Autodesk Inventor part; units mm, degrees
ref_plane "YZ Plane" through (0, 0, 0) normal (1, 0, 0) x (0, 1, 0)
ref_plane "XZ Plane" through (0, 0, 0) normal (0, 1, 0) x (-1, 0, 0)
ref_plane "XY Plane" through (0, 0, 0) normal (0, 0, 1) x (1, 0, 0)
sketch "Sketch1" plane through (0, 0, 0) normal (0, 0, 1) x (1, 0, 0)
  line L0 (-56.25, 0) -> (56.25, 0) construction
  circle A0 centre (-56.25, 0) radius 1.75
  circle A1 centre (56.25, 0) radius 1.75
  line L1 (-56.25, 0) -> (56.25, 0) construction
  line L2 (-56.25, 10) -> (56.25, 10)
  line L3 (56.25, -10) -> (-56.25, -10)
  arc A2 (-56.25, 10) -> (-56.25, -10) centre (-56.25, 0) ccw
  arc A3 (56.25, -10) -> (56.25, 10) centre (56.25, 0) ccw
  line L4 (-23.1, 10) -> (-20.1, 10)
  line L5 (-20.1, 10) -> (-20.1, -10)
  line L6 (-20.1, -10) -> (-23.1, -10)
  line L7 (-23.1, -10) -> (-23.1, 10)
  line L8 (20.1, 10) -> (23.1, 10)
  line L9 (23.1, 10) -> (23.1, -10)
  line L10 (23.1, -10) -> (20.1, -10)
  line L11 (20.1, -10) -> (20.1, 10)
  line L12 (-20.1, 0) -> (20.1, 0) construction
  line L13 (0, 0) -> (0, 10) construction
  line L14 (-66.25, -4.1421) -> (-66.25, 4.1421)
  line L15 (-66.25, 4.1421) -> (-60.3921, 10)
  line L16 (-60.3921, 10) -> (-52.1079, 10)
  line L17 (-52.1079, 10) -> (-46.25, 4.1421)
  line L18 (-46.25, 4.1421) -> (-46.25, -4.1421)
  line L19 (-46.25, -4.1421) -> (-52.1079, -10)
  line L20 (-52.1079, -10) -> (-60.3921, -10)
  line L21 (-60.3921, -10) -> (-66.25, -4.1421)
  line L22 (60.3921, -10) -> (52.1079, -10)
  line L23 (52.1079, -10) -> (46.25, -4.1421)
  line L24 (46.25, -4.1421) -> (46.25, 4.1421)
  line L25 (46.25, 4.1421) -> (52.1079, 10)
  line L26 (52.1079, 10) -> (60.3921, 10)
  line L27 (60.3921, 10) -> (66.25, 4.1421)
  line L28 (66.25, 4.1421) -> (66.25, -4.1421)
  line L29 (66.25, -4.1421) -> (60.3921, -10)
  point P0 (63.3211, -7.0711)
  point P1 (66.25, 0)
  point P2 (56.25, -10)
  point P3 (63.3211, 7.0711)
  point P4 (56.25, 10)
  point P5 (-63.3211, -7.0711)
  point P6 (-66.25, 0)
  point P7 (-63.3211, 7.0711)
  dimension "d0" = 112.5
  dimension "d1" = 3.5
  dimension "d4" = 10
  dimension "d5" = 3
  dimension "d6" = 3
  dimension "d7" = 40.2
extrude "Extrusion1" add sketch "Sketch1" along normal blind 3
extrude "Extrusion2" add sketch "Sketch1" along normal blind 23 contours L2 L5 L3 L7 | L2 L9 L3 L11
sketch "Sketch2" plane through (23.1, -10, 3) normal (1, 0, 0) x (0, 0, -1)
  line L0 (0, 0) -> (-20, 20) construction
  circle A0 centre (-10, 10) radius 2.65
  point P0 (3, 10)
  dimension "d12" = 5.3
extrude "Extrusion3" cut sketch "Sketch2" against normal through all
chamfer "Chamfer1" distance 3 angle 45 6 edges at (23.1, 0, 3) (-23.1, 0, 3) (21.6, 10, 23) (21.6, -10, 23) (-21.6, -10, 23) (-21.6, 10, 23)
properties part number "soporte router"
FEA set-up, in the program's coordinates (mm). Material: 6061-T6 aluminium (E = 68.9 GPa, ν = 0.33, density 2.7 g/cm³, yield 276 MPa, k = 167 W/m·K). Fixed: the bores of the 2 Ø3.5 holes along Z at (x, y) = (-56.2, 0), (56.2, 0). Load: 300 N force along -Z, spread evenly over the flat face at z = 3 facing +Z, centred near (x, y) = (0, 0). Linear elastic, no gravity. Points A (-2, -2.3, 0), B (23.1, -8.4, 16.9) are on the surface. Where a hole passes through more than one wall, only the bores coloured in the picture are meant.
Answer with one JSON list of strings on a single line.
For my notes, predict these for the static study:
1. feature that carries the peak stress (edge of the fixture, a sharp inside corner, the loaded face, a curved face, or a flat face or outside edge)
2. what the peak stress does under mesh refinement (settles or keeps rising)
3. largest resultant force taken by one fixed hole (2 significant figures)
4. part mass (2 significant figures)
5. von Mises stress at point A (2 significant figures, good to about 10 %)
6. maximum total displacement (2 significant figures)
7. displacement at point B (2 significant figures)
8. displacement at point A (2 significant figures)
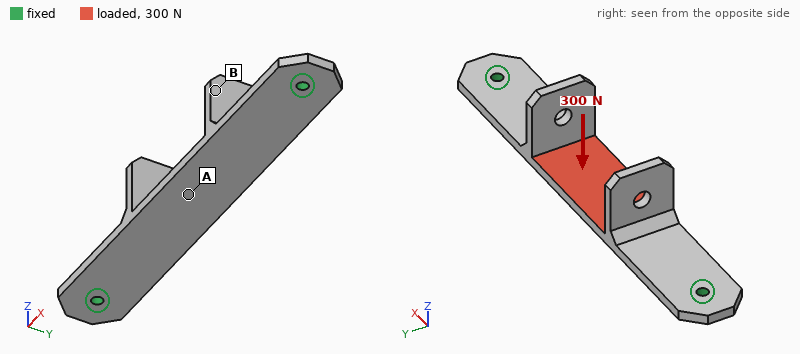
["edge of the fixture", "keeps rising", "150 N", "27 g", "94 MPa", "0.64 mm", "0.48 mm", "0.63 mm"]
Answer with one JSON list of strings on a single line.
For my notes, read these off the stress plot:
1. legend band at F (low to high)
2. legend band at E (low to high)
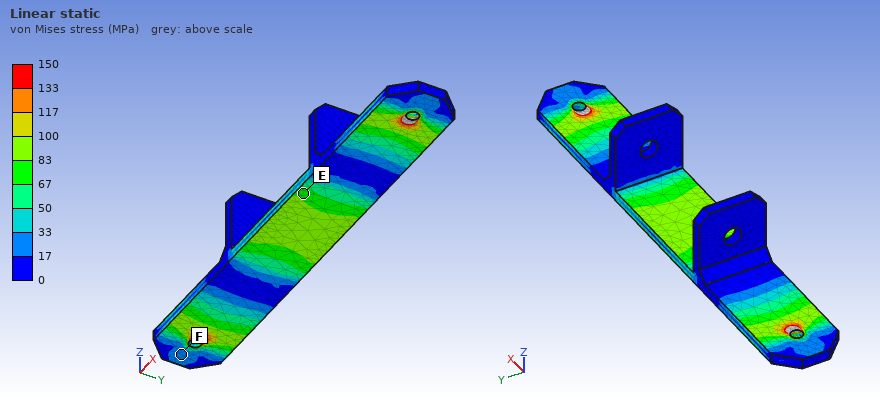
["17 to 33 MPa", "67 to 83 MPa"]
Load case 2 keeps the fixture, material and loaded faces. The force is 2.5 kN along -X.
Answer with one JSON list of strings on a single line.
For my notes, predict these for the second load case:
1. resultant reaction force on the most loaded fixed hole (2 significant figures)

["1.3 kN"]
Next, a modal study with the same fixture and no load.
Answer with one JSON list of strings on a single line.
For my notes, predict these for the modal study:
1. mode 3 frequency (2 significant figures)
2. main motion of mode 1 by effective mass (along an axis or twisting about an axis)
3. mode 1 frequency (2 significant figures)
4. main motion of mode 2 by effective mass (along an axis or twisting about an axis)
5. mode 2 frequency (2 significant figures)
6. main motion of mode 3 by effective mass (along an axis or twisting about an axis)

["2700 Hz", "along Z", "1000 Hz", "along Y", "2100 Hz", "twisting about Y"]
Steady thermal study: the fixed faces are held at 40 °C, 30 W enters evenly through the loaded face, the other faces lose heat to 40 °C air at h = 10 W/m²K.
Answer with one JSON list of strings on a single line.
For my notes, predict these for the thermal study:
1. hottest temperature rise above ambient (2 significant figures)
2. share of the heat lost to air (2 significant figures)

["66 K", "8.0 %"]
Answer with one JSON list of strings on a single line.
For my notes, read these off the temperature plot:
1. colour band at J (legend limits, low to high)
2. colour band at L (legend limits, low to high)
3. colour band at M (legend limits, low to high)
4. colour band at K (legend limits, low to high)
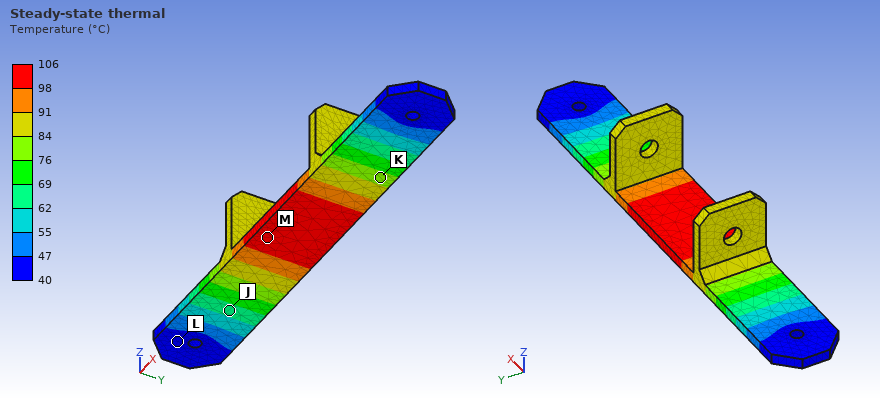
["62 to 69 °C", "40 to 47 °C", "98 to 106 °C", "76 to 84 °C"]
